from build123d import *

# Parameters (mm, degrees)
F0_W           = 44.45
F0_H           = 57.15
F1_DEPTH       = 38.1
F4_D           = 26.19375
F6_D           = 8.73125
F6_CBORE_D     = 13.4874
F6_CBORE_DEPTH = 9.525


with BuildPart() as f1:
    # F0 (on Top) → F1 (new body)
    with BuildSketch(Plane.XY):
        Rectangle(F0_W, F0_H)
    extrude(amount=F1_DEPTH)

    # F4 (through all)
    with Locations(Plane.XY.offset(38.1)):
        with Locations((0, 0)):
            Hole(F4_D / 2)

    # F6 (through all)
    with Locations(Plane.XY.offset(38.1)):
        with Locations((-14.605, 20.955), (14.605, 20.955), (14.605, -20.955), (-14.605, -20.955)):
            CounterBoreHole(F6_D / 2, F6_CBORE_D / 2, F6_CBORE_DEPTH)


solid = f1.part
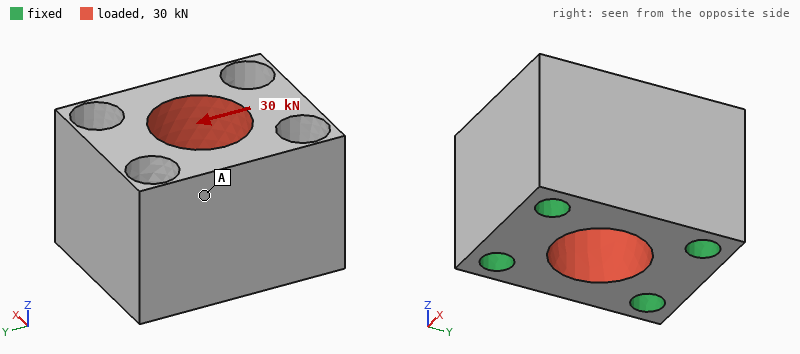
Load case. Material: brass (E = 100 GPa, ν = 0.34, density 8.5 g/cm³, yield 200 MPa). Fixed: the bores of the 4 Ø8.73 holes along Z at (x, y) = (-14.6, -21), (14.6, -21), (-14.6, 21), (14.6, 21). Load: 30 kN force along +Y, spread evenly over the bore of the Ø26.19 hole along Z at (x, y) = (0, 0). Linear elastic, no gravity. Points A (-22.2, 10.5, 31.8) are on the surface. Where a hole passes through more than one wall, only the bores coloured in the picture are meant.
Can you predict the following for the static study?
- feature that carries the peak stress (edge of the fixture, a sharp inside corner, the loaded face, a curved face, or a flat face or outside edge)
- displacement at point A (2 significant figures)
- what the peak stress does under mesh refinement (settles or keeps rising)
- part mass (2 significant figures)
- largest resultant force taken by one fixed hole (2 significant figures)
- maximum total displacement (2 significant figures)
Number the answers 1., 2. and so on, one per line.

1. edge of the fixture
2. 1.6 µm
3. keeps rising
4. 540 g
5. 7.7 kN
6. 5.5 µm
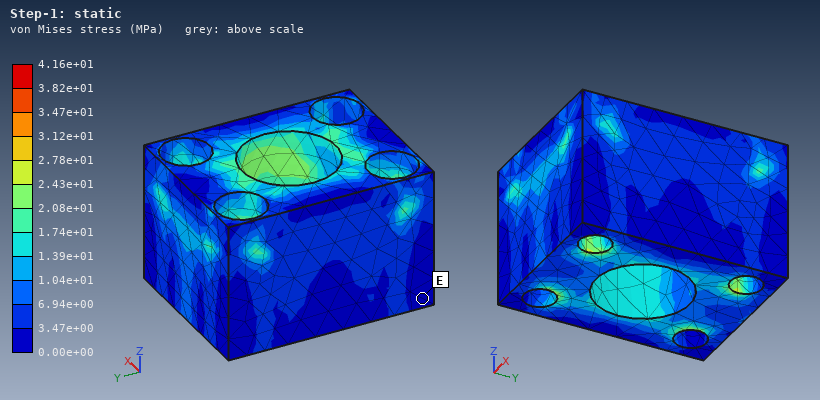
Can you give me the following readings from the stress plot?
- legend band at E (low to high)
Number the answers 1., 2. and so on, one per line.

1. 0.00e+00 to 3.47e+00 MPa
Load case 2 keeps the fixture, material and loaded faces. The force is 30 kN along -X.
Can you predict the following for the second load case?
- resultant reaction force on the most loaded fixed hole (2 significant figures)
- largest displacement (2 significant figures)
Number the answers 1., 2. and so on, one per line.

1. 7.8 kN
2. 8.8 µm
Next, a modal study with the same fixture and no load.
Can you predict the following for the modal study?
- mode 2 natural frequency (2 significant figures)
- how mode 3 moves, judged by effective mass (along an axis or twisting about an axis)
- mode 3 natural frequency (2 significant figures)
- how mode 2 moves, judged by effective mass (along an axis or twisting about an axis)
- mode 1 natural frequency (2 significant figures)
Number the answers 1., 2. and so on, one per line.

1. 21 kHz
2. along Y
3. 25 kHz
4. along X
5. 20 kHz
